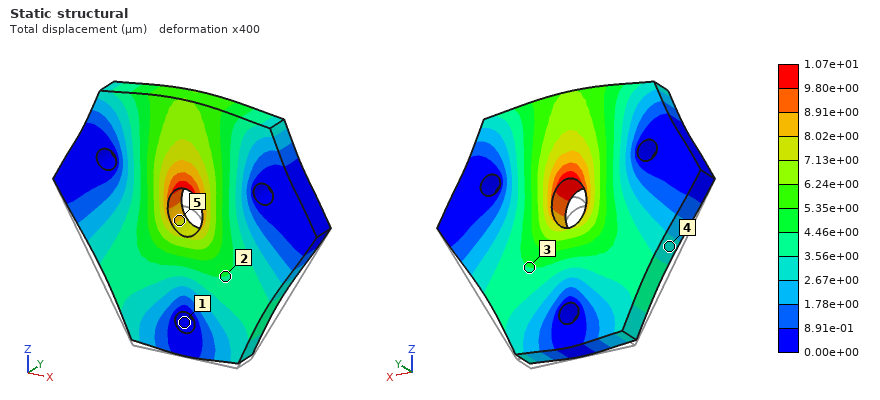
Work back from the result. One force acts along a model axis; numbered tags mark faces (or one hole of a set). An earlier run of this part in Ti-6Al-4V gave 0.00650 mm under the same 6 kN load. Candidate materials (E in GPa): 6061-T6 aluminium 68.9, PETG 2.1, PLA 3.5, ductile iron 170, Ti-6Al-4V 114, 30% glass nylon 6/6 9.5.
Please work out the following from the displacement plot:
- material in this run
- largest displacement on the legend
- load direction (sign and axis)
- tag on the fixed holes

6061-T6 aluminium
1.07e+01 µm
+Z
1
